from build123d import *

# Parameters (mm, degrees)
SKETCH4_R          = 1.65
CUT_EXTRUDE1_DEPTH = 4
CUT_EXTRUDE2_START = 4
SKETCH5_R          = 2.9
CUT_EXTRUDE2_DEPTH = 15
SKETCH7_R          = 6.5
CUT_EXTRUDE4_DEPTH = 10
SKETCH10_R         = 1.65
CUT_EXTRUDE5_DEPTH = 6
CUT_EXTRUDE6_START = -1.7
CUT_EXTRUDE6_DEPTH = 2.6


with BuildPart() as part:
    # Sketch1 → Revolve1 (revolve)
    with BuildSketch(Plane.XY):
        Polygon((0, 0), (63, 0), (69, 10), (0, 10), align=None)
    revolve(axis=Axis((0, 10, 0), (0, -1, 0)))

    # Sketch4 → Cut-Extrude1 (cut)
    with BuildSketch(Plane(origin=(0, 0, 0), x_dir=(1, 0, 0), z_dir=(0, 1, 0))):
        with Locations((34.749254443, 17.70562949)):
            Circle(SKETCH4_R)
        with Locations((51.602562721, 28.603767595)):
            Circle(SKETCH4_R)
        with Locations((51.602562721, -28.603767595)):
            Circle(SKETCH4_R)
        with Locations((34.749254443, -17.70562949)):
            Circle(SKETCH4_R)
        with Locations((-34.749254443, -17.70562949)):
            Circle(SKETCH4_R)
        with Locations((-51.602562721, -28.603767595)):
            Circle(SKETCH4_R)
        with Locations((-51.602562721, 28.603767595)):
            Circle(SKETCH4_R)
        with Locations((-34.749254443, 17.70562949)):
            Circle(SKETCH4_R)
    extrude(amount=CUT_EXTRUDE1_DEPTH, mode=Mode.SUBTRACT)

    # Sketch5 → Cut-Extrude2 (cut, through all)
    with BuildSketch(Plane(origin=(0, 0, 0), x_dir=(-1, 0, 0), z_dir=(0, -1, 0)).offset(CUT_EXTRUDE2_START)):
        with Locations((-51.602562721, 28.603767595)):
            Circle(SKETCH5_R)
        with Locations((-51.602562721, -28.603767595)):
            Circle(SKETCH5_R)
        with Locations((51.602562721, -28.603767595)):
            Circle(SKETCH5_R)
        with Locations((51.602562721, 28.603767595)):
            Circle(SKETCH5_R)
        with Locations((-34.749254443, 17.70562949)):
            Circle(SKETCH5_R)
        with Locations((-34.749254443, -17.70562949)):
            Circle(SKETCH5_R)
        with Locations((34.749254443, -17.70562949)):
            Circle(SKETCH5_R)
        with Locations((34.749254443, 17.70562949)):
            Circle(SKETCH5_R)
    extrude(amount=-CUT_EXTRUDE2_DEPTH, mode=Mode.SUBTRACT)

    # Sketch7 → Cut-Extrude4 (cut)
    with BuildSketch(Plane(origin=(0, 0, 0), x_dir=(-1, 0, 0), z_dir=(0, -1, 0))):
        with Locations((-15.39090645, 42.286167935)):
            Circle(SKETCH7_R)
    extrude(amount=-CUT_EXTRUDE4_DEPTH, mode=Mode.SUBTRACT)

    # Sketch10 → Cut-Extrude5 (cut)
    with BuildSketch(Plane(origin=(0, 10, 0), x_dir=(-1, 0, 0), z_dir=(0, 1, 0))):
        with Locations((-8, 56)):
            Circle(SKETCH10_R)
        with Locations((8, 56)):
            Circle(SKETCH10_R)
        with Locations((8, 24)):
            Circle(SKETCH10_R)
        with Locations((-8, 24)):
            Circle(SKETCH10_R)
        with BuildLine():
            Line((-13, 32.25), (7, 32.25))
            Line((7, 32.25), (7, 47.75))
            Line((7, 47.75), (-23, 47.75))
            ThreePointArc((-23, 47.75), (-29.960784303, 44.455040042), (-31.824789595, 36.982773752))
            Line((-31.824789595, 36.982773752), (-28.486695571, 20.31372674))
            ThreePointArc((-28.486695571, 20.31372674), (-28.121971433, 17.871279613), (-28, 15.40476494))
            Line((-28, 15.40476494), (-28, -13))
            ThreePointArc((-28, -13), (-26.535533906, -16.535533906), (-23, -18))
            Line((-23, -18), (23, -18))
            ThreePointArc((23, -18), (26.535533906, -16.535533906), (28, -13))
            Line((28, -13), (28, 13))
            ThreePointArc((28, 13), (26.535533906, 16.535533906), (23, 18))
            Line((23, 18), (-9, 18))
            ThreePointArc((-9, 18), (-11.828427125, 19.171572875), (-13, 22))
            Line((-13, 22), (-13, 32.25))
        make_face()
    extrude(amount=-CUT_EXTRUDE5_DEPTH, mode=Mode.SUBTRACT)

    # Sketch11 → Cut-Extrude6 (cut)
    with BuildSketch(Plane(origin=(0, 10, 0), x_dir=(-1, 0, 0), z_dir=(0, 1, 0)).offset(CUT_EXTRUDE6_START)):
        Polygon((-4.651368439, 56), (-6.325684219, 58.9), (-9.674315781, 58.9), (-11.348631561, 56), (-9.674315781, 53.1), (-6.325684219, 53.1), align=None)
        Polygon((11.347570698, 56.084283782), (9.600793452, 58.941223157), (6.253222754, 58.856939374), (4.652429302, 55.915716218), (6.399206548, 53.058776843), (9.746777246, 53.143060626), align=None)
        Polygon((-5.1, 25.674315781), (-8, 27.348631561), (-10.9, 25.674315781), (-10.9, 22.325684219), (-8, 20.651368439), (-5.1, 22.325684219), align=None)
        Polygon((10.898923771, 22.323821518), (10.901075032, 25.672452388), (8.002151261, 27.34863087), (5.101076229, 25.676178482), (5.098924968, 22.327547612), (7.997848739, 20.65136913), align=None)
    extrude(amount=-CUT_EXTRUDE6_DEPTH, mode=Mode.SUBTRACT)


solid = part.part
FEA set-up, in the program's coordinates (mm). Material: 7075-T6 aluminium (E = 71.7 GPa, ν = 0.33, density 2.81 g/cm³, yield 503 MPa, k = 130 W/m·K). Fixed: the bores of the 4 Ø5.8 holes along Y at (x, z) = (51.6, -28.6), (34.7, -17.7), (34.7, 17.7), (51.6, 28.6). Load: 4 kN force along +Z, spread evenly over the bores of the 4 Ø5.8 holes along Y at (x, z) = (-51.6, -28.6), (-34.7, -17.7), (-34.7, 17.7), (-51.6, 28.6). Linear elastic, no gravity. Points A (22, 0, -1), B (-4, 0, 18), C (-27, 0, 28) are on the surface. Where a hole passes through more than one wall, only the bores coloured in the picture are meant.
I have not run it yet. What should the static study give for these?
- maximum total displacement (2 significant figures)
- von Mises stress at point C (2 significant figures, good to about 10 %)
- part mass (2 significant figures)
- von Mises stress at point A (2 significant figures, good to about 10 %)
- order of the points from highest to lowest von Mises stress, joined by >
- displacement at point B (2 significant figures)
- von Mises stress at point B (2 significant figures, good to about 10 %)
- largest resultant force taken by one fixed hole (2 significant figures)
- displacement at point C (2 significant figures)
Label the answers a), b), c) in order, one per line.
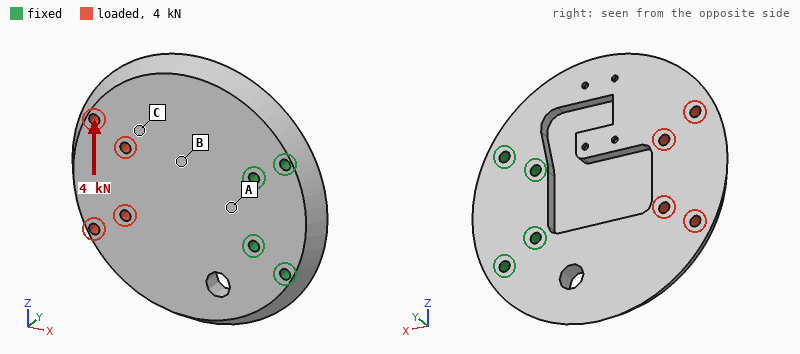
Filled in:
a) 0.10 mm
b) 5.8 MPa
c) 330 g
d) 31 MPa
e) A > B > C
f) 0.028 mm
g) 15 MPa
h) 4.2 kN
i) 0.046 mm
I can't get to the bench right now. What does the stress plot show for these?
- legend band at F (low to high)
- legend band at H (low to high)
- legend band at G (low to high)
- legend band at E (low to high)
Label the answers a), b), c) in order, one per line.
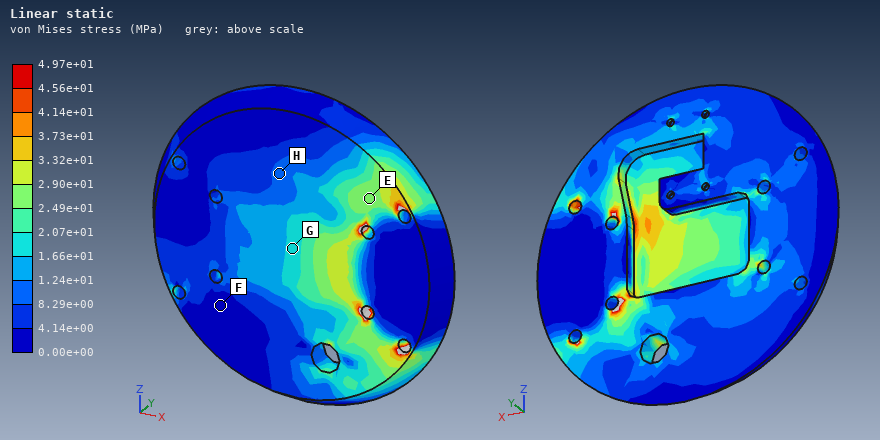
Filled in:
a) 0.00e+00 to 4.14e+00 MPa
b) 8.29e+00 to 1.24e+01 MPa
c) 1.66e+01 to 2.07e+01 MPa
d) 2.49e+01 to 2.90e+01 MPa
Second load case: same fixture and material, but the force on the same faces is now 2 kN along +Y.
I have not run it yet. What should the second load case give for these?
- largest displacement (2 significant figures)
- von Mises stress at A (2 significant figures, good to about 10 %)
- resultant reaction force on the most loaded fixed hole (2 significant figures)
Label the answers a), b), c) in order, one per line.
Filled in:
a) 1.5 mm
b) 110 MPa
c) 3.9 kN
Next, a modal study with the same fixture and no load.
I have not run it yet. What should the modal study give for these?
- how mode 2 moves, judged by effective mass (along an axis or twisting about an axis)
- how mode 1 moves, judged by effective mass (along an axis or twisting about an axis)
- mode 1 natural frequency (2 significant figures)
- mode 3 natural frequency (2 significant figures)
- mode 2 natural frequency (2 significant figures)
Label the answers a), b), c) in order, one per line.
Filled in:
a) twisting about X
b) along Y
c) 640 Hz
d) 2900 Hz
e) 1300 Hz
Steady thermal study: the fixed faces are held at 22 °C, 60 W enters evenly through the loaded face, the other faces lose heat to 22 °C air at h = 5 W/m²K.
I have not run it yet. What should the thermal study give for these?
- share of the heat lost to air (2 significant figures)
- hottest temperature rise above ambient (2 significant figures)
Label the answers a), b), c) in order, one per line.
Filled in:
a) 6.7 %
b) 50 K
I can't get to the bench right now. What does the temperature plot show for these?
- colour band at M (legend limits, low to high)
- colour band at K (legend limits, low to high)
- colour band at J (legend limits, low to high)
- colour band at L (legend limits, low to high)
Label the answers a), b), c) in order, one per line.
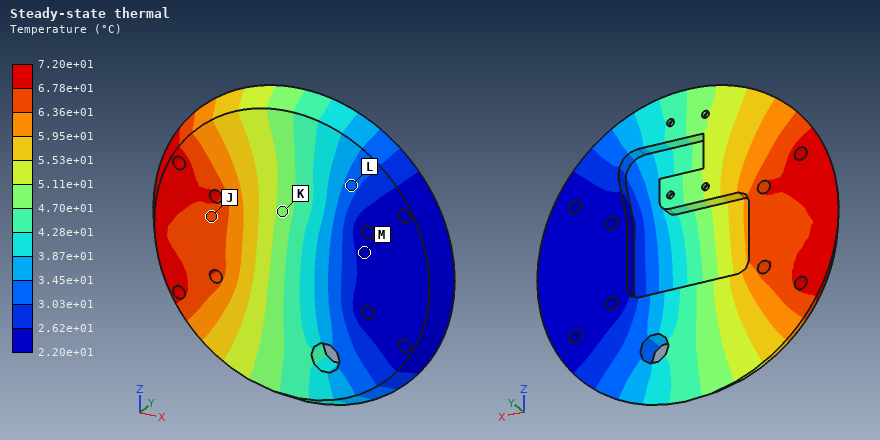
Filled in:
a) 2.20e+01 to 2.62e+01 °C
b) 4.70e+01 to 5.11e+01 °C
c) 6.36e+01 to 6.78e+01 °C
d) 3.03e+01 to 3.45e+01 °C
